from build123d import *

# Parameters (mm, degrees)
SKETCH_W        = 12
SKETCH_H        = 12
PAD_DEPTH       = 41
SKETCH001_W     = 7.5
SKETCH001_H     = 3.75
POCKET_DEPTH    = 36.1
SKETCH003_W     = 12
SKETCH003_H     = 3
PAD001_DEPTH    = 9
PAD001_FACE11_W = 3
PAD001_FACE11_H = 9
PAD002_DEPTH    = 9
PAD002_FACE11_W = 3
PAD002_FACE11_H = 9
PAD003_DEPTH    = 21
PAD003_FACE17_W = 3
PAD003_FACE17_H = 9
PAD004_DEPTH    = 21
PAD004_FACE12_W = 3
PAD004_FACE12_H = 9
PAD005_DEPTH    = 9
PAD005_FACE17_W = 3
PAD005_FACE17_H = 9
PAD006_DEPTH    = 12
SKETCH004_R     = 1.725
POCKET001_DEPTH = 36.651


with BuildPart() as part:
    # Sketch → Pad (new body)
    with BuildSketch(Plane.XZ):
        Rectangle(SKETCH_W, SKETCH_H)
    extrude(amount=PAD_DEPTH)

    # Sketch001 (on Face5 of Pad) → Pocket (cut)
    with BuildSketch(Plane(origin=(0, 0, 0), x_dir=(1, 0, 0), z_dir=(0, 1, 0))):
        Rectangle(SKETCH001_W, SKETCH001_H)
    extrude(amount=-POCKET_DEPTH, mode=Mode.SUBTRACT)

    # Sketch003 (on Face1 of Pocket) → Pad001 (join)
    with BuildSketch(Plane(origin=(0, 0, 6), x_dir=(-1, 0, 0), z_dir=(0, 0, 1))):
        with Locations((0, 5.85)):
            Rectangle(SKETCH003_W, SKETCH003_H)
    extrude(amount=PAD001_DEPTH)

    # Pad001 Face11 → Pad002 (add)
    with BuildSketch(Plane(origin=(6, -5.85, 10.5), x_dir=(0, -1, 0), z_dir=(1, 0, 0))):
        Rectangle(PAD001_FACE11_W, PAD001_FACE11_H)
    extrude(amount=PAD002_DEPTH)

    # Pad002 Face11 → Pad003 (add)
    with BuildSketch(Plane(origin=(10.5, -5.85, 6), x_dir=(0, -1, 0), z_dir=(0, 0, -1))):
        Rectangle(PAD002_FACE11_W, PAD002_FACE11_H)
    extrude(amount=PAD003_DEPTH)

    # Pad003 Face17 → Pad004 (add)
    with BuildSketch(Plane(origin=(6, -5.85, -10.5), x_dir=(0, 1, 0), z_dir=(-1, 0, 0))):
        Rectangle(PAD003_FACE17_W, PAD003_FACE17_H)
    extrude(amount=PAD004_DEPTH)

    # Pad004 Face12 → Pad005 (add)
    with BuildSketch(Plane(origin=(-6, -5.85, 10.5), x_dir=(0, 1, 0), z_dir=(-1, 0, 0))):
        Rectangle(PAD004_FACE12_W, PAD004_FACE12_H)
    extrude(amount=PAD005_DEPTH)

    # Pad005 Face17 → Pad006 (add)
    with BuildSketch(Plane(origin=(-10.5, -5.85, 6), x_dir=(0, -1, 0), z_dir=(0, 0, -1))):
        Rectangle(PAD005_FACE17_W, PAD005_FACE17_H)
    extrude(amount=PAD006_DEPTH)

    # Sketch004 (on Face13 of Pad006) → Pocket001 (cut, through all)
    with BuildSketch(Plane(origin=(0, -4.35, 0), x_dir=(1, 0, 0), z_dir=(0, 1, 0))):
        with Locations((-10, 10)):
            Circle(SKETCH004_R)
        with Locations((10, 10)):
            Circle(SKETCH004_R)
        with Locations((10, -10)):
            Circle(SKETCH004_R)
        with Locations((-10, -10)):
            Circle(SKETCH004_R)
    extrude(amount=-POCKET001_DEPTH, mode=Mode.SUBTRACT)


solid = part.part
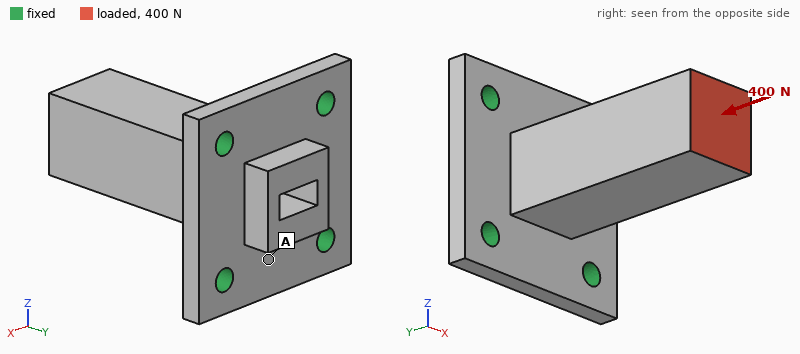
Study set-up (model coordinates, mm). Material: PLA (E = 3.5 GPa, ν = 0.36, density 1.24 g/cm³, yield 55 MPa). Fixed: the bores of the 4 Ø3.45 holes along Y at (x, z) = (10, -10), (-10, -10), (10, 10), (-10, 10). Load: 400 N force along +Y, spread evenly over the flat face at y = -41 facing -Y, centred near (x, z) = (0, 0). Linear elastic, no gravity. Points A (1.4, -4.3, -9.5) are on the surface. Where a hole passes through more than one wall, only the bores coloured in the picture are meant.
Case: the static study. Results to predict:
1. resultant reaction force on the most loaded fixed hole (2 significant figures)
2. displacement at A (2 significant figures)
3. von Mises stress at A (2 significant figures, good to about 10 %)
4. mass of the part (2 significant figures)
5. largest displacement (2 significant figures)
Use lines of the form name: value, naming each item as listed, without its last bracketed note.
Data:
resultant reaction force on the most loaded fixed hole: 100 N
displacement at A: 35 µm
von Mises stress at A: 4.8 MPa
mass of the part: 8.7 g
largest displacement: 86 µm
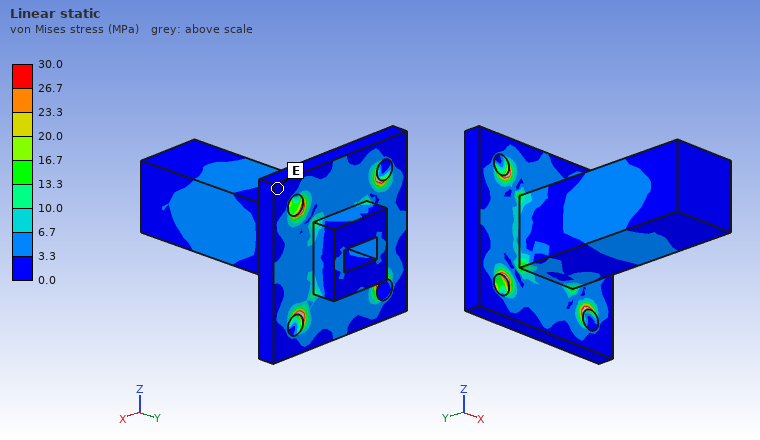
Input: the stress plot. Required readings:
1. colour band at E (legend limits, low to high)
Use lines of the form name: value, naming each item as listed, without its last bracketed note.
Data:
colour band at E: 0.0 to 3.3 MPa
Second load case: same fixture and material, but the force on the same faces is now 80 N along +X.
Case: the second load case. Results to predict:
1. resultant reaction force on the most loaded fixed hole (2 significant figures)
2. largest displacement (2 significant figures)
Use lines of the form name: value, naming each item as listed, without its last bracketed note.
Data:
resultant reaction force on the most loaded fixed hole: 87 N
largest displacement: 0.44 mm
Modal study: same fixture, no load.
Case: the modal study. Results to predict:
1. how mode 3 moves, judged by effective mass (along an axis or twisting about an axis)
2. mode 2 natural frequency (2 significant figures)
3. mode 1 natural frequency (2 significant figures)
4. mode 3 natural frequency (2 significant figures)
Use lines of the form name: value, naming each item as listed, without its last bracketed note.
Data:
how mode 3 moves, judged by effective mass: along Y
mode 2 natural frequency: 1700 Hz
mode 1 natural frequency: 1700 Hz
mode 3 natural frequency: 5100 Hz
